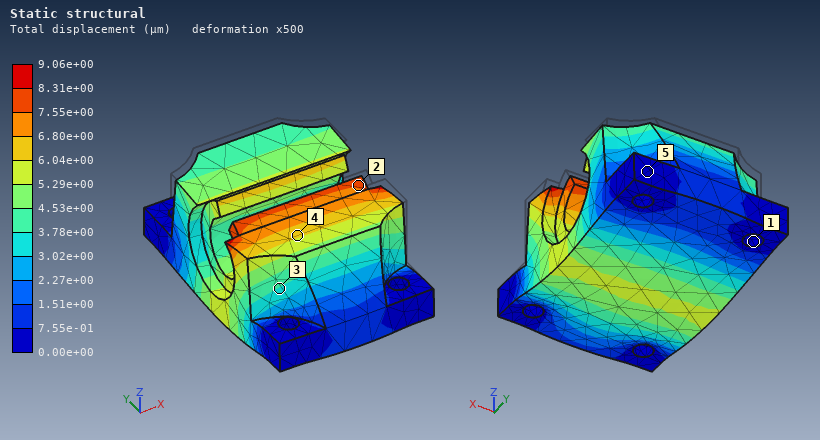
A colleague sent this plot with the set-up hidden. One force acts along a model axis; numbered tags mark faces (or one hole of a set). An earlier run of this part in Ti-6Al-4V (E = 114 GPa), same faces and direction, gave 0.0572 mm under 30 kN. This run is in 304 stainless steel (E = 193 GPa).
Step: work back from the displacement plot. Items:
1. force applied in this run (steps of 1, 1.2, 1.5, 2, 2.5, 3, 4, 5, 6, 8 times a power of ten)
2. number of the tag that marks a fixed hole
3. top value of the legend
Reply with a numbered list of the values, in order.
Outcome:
1. 8 kN
2. 1
3. 9.06e+00 µm
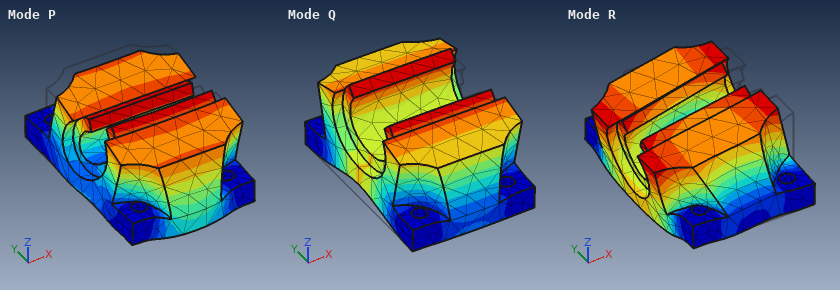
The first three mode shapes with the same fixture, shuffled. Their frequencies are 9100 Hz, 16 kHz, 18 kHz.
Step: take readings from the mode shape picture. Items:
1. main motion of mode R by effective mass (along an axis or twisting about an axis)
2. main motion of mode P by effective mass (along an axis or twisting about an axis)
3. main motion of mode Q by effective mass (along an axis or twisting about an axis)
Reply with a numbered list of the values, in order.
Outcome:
1. along X
2. along Y
3. along Z
